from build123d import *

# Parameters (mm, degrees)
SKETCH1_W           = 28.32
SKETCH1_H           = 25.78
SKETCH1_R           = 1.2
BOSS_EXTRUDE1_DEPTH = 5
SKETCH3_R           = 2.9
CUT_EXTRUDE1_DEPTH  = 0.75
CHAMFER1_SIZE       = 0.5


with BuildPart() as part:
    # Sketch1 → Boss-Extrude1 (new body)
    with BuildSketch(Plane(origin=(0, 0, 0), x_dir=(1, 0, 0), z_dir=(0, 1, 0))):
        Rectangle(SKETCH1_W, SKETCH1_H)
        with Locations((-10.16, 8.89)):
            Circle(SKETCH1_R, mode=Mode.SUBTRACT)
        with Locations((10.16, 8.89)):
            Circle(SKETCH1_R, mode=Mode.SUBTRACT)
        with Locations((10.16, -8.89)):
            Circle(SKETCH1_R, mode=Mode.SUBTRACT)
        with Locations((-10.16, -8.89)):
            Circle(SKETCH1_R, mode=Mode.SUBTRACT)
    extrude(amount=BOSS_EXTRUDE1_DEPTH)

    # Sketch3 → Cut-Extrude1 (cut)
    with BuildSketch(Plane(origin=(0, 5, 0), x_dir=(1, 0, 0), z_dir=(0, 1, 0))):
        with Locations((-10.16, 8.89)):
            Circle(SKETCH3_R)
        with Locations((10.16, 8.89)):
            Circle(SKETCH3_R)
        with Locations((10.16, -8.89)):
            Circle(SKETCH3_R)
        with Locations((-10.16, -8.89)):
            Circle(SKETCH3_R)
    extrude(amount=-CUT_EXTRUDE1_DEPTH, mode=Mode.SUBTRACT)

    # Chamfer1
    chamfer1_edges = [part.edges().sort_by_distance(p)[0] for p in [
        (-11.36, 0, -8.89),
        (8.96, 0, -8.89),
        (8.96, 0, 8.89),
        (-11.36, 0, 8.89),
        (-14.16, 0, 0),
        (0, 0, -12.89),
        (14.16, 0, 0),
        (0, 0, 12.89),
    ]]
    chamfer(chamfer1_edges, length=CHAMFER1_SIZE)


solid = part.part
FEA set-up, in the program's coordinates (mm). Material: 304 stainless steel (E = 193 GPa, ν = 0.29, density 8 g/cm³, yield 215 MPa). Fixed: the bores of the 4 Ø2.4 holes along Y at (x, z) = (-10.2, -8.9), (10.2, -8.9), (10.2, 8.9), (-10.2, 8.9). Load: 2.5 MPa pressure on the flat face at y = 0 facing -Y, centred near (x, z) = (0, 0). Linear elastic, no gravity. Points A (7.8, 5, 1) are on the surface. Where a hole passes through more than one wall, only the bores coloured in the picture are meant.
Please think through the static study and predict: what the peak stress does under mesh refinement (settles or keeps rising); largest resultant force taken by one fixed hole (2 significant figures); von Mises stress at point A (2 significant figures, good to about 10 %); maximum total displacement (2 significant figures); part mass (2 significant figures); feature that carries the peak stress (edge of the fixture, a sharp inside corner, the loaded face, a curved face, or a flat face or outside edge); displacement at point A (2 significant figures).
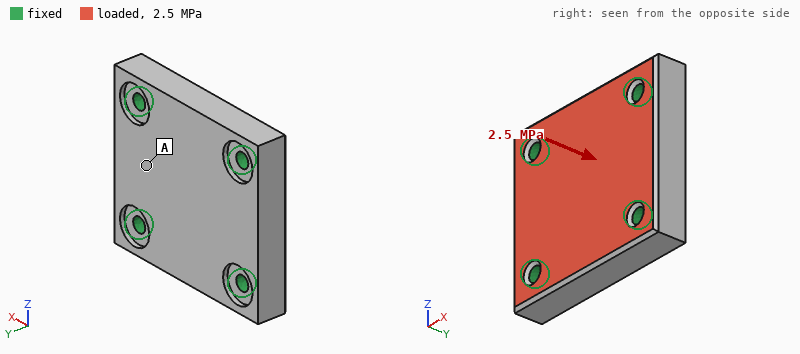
keeps rising
400 N
10 MPa
1.9 µm
28 g
edge of the fixture
1.3 µm
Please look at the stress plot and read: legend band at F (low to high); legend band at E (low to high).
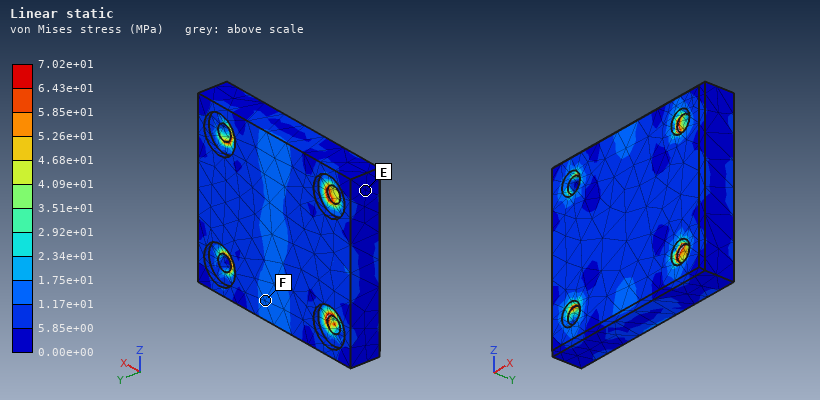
1.17e+01 to 1.75e+01 MPa
0.00e+00 to 5.85e+00 MPa
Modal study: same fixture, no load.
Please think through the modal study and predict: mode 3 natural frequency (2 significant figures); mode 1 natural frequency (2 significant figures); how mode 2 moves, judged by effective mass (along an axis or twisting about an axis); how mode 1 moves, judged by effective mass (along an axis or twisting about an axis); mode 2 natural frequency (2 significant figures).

51 kHz
34 kHz
twisting about X
along Y
45 kHz
